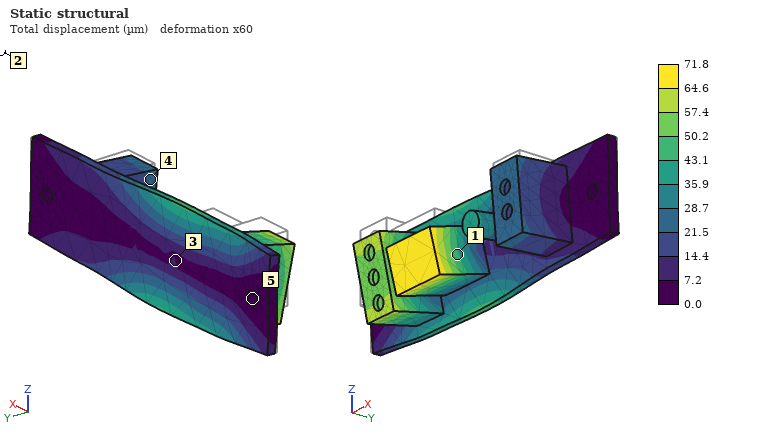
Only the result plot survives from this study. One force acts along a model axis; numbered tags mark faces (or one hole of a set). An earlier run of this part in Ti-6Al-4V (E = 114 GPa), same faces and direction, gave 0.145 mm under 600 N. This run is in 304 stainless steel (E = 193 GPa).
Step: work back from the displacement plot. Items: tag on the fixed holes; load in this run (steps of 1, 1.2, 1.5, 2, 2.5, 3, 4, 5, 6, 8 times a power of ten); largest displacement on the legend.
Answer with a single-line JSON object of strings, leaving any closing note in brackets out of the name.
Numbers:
{"tag on the fixed holes": "5", "load in this run": "500 N", "largest displacement on the legend": "71.8 µm"}
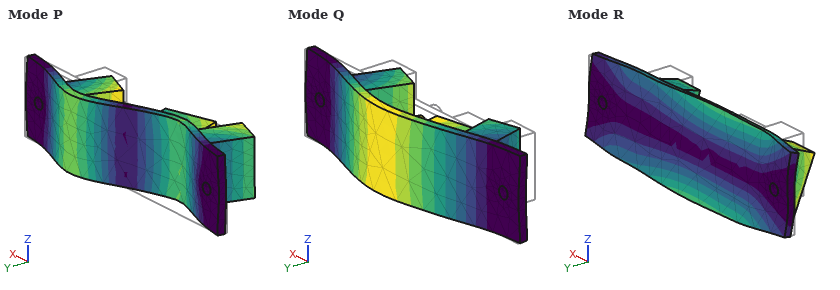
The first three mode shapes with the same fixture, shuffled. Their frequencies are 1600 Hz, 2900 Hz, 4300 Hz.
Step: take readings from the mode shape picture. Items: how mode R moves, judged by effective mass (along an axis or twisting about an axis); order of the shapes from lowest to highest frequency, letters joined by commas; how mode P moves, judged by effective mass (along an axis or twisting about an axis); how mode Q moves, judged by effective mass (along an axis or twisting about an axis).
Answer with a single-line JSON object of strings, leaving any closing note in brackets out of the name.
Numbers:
{"how mode R moves, judged by effective mass": "along Z", "order of the shapes from lowest to highest frequency, letters joined by commas": "Q, R, P", "how mode P moves, judged by effective mass": "twisting about Z", "how mode Q moves, judged by effective mass": "along Y"}
